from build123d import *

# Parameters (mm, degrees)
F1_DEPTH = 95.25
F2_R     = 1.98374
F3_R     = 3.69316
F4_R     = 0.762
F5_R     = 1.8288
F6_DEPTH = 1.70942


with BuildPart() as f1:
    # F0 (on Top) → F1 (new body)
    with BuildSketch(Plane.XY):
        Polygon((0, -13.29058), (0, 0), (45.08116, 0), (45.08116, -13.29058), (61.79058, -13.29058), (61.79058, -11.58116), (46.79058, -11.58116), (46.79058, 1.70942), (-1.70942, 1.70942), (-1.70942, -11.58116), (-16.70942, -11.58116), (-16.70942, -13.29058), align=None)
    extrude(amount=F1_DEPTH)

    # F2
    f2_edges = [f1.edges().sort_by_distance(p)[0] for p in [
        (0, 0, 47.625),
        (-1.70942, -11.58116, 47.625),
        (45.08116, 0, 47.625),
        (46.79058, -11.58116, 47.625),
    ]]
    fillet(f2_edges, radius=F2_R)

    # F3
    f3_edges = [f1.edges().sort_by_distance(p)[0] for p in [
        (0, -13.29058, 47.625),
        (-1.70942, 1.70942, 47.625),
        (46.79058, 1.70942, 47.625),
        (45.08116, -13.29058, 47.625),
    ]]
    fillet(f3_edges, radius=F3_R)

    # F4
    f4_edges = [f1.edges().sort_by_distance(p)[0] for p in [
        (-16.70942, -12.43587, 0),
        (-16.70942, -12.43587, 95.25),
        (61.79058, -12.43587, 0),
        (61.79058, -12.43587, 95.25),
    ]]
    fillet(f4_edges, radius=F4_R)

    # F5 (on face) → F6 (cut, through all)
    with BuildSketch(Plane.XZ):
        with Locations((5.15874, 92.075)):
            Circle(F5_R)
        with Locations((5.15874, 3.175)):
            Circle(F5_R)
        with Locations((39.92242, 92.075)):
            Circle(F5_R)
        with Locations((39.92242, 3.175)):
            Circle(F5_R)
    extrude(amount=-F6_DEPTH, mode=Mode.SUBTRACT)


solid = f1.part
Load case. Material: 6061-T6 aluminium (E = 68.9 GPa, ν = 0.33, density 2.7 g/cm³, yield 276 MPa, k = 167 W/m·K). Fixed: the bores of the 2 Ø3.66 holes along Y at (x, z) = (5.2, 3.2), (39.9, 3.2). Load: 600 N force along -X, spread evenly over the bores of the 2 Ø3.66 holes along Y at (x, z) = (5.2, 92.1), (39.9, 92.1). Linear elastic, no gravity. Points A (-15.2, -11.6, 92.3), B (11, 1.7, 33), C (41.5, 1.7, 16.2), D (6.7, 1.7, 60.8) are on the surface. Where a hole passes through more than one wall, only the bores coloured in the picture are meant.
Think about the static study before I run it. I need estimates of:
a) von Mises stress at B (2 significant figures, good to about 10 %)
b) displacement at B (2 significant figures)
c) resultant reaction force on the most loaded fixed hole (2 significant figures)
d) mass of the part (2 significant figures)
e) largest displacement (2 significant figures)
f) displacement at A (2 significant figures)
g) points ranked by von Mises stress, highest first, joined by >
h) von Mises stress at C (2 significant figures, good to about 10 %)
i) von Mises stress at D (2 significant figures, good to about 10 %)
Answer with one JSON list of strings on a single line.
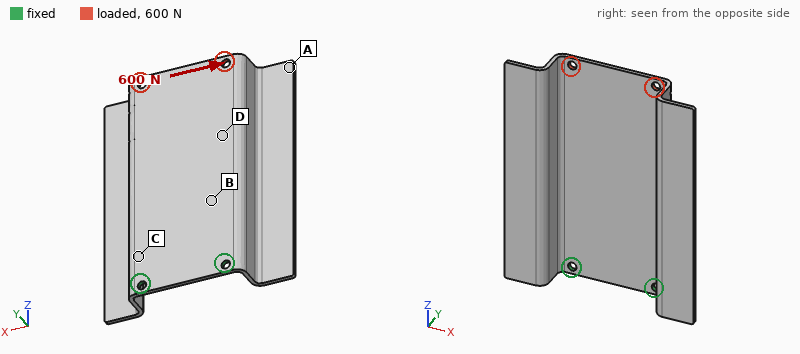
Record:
["26 MPa", "0.038 mm", "1.5 kN", "44 g", "0.21 mm", "0.20 mm", "C > B > D > A", "51 MPa", "17 MPa"]
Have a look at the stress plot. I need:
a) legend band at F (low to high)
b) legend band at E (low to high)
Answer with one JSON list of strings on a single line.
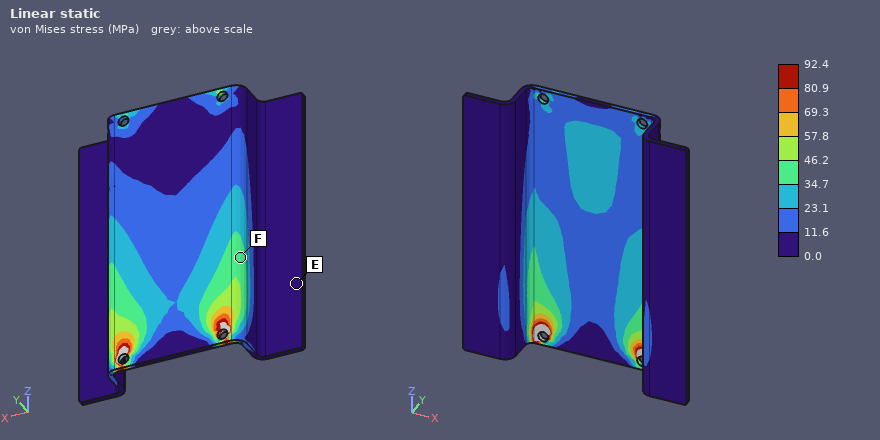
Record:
["34.7 to 46.2 MPa", "0.0 to 11.6 MPa"]
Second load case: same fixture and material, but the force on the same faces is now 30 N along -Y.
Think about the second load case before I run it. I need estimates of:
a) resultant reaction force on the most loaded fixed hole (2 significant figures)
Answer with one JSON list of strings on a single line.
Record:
["51 N"]
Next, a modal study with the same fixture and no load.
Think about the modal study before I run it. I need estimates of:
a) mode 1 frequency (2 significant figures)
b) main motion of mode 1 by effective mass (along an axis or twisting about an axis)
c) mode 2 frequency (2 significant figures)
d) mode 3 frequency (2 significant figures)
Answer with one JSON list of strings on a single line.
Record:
["280 Hz", "along Y", "400 Hz", "1100 Hz"]
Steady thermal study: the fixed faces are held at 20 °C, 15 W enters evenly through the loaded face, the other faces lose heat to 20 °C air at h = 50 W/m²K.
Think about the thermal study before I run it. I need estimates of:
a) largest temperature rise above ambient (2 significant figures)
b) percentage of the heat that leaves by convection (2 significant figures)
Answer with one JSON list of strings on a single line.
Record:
["38 K", "74 %"]
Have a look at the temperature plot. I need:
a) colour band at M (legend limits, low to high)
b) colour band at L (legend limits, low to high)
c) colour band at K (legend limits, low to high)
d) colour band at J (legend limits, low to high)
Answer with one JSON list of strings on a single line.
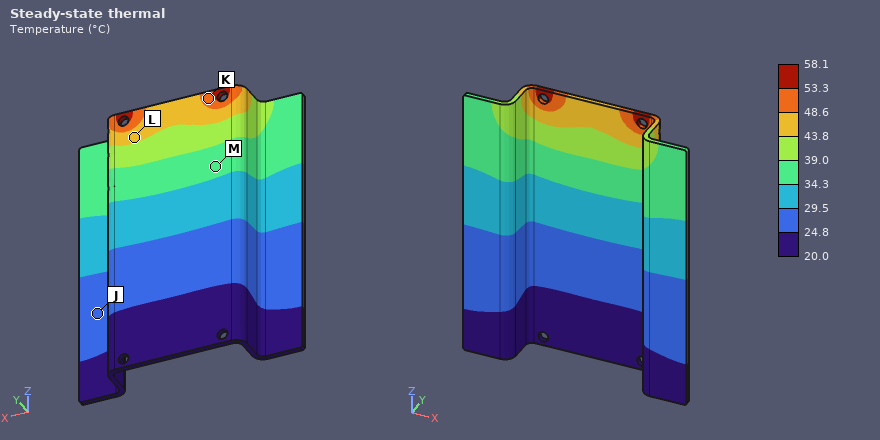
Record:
["34.3 to 39.0 °C", "43.8 to 48.6 °C", "48.6 to 53.3 °C", "24.8 to 29.5 °C"]
